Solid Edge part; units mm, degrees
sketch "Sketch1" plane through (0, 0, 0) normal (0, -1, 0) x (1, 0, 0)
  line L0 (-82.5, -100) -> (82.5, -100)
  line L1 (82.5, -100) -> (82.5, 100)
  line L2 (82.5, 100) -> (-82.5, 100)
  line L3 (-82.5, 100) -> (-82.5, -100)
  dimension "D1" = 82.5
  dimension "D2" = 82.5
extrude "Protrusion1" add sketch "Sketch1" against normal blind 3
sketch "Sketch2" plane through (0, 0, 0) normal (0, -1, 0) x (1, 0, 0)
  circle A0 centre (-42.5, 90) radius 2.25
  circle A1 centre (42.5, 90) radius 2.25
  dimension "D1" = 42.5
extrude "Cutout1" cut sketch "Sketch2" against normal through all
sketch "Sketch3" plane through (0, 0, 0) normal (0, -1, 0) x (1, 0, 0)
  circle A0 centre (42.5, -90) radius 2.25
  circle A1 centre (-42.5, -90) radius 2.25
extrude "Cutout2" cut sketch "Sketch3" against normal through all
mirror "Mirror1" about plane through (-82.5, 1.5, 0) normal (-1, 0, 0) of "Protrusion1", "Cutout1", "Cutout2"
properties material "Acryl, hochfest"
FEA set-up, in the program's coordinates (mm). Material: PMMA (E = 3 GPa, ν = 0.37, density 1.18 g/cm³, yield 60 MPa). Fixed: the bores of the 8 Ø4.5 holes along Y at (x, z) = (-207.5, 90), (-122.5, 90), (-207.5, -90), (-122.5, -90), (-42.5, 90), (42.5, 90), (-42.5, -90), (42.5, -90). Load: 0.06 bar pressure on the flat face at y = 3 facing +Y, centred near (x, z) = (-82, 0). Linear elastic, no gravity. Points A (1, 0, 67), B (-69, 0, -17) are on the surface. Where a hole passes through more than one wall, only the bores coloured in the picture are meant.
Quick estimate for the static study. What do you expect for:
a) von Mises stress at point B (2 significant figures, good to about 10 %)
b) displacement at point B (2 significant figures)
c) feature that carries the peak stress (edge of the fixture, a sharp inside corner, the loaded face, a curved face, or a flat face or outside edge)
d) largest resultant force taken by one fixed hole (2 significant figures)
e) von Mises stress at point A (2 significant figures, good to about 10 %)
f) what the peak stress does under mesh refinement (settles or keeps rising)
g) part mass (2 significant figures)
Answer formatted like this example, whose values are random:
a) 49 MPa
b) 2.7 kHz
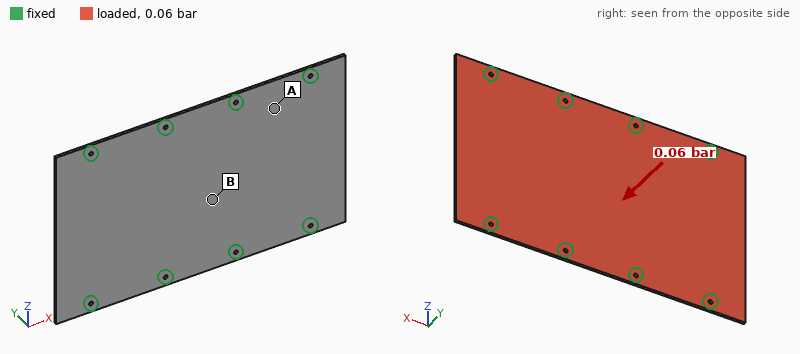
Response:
a) 5.2 MPa
b) 2.9 mm
c) edge of the fixture
d) 51 N
e) 2.0 MPa
f) keeps rising
g) 230 g
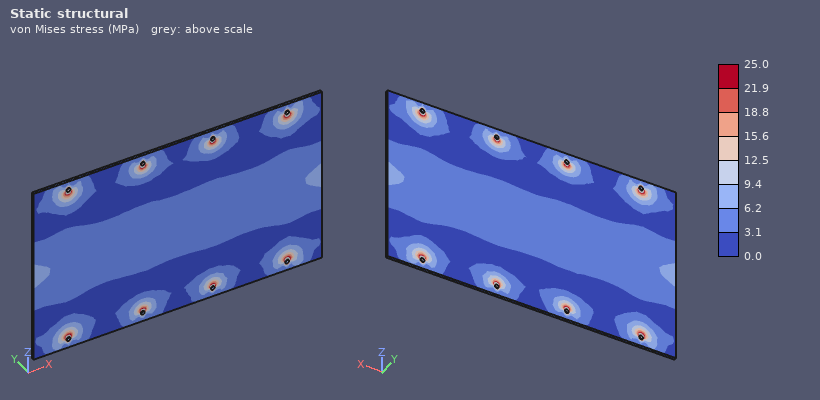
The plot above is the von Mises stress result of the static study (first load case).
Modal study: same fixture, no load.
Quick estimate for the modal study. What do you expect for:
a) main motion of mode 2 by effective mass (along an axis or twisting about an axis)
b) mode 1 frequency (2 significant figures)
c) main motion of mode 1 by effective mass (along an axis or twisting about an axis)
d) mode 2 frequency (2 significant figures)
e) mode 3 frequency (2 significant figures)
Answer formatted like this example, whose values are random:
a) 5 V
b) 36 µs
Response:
a) twisting about Z
b) 130 Hz
c) along Y
d) 140 Hz
e) 170 Hz
